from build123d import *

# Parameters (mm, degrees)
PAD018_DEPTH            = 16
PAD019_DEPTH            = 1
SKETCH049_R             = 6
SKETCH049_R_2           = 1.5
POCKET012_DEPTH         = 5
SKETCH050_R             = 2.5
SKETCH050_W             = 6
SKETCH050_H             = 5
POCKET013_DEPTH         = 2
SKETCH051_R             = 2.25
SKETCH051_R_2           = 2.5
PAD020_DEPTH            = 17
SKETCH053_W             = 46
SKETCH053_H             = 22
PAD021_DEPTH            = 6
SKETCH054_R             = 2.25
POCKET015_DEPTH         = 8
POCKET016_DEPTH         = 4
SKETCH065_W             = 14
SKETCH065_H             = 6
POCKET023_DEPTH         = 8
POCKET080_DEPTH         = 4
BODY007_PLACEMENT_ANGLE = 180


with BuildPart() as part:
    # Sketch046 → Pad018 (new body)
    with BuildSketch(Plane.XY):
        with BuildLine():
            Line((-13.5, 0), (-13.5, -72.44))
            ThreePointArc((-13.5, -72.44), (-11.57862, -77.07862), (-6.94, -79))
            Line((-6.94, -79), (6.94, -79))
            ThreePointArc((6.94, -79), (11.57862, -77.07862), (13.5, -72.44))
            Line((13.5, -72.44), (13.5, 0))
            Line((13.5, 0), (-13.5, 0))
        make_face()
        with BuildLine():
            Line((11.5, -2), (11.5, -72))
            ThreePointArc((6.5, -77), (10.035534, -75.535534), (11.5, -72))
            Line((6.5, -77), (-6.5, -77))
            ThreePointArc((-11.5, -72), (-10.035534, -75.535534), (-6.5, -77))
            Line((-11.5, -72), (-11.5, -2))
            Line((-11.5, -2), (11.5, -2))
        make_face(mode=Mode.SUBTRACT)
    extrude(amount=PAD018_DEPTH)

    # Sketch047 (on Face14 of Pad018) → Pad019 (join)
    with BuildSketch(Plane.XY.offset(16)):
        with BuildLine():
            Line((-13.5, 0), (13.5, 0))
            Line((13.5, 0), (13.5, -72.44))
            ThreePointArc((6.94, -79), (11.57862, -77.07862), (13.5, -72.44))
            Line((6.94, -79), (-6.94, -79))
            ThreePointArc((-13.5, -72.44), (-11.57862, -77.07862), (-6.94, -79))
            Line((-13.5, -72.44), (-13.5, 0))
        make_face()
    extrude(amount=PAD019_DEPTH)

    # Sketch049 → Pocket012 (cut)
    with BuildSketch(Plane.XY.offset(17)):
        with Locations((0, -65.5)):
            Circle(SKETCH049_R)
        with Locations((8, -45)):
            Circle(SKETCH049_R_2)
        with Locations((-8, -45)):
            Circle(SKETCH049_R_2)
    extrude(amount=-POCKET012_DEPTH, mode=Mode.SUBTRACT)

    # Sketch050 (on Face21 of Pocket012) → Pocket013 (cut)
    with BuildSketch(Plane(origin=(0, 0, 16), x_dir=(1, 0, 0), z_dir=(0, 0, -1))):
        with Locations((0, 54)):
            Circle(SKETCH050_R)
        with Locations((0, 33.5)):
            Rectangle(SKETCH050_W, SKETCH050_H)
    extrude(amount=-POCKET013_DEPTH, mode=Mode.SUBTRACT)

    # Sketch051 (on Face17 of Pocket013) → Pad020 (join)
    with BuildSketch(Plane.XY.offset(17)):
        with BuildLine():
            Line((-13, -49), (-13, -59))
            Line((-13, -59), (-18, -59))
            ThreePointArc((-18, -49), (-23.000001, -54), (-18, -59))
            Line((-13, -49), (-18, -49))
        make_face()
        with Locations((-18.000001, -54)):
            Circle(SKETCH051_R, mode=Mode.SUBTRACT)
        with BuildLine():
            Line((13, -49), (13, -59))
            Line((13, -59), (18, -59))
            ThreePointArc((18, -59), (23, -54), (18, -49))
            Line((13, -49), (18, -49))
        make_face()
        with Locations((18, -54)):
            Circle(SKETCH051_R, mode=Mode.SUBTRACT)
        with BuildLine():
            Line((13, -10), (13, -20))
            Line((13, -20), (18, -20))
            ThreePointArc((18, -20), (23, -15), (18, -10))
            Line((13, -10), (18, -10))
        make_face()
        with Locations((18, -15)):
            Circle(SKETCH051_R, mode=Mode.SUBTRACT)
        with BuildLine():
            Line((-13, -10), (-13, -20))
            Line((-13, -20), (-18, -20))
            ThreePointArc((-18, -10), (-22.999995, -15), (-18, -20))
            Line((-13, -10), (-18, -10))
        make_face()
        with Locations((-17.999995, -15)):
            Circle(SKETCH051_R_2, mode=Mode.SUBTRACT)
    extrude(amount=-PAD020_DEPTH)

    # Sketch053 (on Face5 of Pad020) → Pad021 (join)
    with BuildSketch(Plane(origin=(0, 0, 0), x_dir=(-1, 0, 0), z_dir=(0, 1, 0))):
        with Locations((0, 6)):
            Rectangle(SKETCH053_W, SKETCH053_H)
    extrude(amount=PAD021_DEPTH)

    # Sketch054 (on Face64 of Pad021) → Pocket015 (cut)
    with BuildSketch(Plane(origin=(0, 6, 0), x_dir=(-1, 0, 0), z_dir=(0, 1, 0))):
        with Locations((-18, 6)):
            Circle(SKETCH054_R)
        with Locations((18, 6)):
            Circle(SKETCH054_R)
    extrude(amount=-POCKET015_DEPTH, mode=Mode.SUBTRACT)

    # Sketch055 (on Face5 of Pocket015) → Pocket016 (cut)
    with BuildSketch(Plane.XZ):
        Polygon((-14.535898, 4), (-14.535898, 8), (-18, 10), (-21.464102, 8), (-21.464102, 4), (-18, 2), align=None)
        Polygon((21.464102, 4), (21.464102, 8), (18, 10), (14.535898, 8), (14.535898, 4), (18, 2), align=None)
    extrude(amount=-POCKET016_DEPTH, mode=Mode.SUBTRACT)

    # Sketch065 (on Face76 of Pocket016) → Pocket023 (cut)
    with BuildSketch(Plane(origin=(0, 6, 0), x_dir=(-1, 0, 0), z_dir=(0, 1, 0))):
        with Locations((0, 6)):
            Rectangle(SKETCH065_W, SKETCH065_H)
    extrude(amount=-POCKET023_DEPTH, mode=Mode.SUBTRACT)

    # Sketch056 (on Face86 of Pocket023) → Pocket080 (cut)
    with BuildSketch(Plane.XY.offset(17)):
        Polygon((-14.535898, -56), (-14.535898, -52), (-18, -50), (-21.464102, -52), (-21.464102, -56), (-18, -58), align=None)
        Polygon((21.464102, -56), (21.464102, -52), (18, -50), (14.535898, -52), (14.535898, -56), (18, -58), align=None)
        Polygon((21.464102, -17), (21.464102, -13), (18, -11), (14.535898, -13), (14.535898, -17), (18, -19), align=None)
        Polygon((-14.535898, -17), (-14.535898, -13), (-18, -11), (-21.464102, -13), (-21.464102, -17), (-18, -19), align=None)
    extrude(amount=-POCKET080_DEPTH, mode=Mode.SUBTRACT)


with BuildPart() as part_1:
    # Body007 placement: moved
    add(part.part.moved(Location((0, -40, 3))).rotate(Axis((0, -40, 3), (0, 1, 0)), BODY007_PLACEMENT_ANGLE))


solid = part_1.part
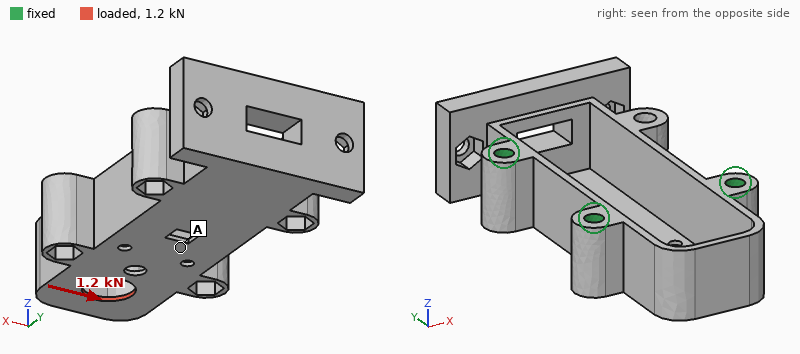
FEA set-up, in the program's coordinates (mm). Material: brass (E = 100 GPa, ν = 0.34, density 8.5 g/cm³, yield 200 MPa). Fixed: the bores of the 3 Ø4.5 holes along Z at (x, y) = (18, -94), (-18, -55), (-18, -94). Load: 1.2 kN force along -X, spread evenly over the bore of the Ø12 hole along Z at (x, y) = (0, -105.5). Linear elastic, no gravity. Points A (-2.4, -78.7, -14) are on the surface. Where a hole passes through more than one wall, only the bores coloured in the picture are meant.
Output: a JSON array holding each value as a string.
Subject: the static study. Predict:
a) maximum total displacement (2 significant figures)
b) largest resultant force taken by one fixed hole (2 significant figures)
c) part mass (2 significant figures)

["34 µm", "710 N", "150 g"]
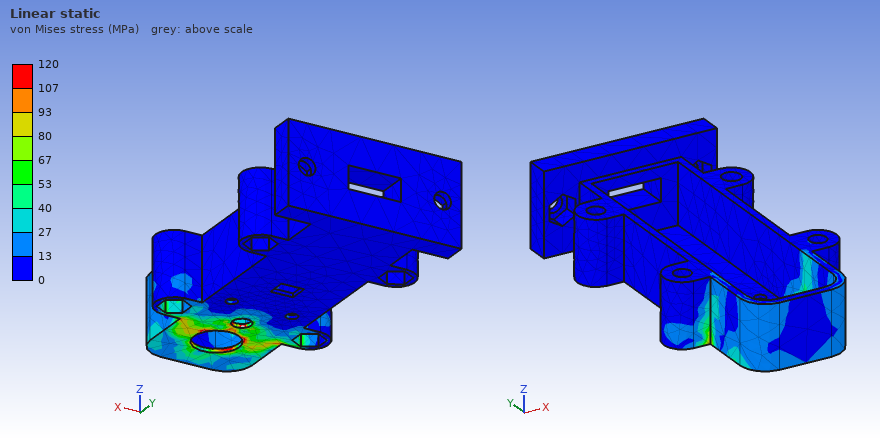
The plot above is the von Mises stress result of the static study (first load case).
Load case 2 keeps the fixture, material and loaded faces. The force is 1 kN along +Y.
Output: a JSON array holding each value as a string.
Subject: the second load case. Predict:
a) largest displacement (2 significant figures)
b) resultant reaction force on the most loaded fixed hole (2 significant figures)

["13 µm", "450 N"]
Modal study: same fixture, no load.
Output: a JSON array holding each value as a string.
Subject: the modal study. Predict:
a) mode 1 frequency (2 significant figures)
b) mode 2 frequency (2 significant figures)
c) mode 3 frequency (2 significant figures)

["1600 Hz", "3500 Hz", "4200 Hz"]
